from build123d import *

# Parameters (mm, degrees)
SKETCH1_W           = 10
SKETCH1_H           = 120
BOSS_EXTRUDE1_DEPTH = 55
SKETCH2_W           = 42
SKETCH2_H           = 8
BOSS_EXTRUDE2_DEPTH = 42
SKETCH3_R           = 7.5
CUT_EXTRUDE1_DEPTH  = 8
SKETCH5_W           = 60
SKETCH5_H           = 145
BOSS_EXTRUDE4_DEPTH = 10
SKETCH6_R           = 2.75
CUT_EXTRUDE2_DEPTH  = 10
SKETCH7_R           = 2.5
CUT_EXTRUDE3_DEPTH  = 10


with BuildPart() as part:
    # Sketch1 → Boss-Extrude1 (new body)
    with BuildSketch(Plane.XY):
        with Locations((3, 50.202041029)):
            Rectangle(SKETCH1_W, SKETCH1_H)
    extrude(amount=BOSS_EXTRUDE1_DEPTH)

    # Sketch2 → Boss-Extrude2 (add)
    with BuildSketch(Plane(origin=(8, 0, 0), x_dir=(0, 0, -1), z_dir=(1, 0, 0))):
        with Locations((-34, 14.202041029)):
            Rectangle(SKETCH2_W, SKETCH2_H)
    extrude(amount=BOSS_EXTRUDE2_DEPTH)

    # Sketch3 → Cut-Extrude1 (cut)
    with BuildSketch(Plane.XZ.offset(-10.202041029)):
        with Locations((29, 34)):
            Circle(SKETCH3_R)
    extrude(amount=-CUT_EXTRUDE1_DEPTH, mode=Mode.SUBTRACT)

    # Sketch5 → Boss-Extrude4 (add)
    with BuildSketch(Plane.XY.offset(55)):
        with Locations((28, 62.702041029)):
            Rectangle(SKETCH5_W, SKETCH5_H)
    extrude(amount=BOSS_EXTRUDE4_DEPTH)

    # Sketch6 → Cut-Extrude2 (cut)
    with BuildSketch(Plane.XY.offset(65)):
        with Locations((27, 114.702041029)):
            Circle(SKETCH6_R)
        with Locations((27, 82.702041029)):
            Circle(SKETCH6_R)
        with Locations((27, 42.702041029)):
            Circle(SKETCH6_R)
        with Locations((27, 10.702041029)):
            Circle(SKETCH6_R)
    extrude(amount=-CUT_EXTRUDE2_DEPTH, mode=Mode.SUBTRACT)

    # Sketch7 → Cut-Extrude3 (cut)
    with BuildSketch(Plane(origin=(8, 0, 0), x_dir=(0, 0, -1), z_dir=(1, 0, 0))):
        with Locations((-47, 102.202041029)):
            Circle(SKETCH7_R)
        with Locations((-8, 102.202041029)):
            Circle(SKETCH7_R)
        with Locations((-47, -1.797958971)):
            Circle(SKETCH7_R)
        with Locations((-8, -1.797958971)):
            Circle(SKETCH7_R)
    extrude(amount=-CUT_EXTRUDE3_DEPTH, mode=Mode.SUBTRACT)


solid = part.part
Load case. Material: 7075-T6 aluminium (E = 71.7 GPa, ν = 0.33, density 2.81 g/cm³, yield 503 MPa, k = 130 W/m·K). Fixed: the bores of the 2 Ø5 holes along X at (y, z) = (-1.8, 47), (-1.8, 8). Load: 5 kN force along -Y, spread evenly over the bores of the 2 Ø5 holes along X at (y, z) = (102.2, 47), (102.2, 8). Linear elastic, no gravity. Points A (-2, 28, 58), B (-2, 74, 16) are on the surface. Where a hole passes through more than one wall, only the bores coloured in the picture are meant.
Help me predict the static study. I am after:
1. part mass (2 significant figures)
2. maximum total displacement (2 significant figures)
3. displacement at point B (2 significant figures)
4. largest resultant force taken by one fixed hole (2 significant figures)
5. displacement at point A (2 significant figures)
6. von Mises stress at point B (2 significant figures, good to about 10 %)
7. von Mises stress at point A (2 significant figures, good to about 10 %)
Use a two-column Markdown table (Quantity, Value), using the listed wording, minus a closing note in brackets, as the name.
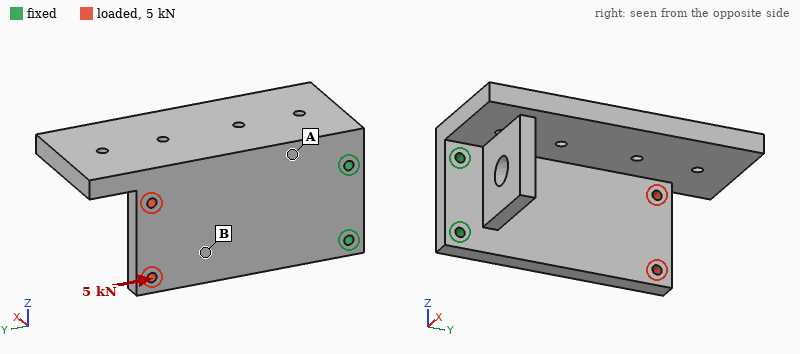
| Quantity | Value |
|---|---|
| part mass | 460 g |
| maximum total displacement | 23 µm |
| displacement at point B | 13 µm |
| largest resultant force taken by one fixed hole | 2.5 kN |
| displacement at point A | 3.7 µm |
| von Mises stress at point B | 9.3 MPa |
| von Mises stress at point A | 4.2 MPa |
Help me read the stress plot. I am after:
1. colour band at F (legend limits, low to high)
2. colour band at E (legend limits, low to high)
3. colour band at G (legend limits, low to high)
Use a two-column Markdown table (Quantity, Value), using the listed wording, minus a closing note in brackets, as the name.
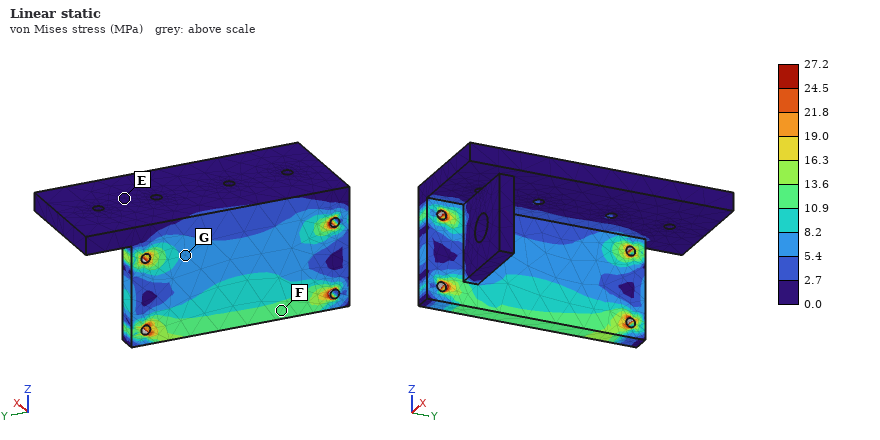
| Quantity | Value |
|---|---|
| colour band at F | 10.9 to 13.6 MPa |
| colour band at E | 0.0 to 2.7 MPa |
| colour band at G | 5.4 to 8.2 MPa |
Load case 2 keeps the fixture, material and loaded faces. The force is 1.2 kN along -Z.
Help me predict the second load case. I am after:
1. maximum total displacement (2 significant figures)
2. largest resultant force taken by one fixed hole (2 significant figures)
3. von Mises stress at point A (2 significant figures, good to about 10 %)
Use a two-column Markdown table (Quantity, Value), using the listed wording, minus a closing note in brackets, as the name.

| Quantity | Value |
|---|---|
| maximum total displacement | 62 µm |
| largest resultant force taken by one fixed hole | 3.1 kN |
| von Mises stress at point A | 7.4 MPa |
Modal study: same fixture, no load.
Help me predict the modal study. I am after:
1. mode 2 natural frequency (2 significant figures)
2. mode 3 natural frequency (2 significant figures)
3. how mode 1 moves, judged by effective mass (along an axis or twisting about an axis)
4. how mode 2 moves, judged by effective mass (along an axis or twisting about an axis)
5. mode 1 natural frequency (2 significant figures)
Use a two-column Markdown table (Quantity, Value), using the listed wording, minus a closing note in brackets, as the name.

| Quantity | Value |
|---|---|
| mode 2 natural frequency | 1200 Hz |
| mode 3 natural frequency | 2200 Hz |
| how mode 1 moves, judged by effective mass | along X |
| how mode 2 moves, judged by effective mass | along Z |
| mode 1 natural frequency | 490 Hz |
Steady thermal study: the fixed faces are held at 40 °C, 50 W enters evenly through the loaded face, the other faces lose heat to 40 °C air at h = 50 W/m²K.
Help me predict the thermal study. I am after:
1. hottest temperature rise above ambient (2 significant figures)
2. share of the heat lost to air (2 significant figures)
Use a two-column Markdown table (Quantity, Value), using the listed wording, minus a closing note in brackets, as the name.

| Quantity | Value |
|---|---|
| hottest temperature rise above ambient | 41 K |
| share of the heat lost to air | 52 % |
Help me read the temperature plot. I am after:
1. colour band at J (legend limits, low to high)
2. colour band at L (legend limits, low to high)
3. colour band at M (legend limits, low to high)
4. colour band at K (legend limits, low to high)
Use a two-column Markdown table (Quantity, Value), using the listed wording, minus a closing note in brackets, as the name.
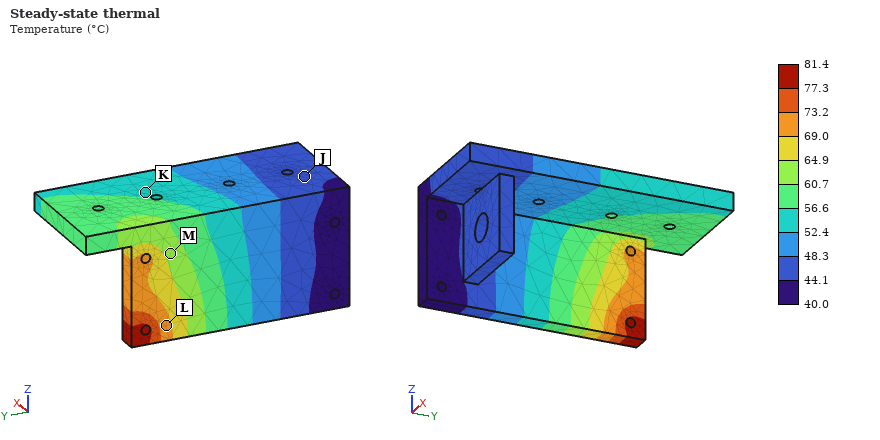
| Quantity | Value |
|---|---|
| colour band at J | 44.1 to 48.3 °C |
| colour band at L | 69.0 to 73.2 °C |
| colour band at M | 60.7 to 64.9 °C |
| colour band at K | 52.4 to 56.6 °C |
